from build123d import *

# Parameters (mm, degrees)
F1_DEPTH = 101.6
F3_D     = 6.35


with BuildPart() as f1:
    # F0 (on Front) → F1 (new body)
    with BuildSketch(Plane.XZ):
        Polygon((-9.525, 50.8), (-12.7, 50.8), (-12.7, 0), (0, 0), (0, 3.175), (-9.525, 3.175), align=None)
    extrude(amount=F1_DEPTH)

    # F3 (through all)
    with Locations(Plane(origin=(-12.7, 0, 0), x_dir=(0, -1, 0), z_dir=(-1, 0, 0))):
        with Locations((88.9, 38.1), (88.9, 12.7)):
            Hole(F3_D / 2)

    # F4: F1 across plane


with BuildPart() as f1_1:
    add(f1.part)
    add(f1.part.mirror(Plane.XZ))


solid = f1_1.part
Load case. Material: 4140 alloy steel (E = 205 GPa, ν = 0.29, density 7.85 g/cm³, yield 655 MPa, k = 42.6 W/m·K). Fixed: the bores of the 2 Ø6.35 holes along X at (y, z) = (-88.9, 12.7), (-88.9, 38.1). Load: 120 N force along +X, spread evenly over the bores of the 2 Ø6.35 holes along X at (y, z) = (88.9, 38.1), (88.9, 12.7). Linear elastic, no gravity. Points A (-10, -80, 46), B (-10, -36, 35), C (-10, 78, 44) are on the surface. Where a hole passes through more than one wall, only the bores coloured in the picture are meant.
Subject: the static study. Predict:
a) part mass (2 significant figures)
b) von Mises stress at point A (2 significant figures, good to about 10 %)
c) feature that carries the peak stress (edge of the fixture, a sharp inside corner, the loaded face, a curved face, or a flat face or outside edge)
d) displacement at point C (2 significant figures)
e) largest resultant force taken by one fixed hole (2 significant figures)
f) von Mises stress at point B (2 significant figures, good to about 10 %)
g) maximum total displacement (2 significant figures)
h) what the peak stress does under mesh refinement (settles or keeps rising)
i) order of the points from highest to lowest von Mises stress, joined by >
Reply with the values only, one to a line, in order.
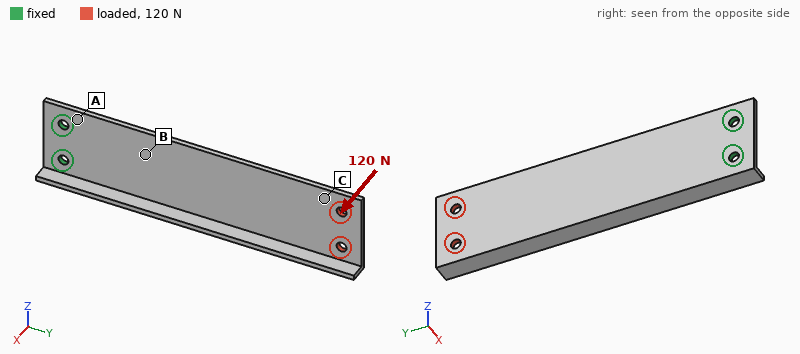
300 g
90 MPa
edge of the fixture
1.7 mm
160 N
31 MPa
2.1 mm
keeps rising
A > B > C
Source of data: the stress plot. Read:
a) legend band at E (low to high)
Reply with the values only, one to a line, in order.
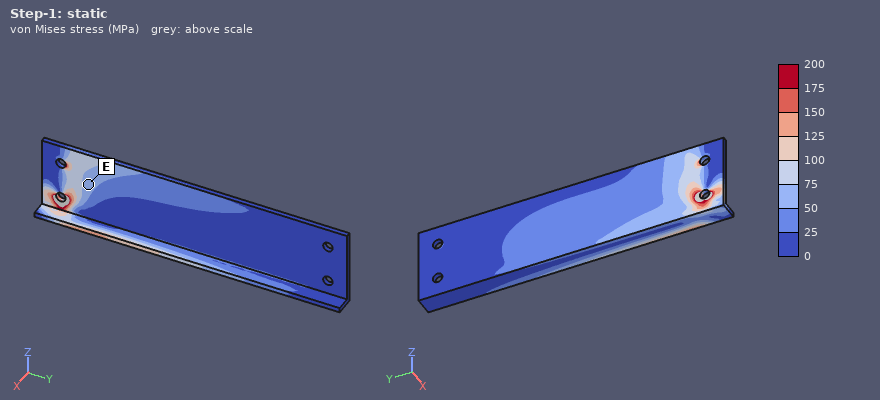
50 to 75 MPa
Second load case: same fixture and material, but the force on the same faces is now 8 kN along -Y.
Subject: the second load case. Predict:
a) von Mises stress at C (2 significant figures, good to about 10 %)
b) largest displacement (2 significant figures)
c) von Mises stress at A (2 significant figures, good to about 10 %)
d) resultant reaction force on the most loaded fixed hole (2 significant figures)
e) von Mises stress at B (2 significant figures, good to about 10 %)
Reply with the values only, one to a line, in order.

49 MPa
0.40 mm
41 MPa
4.0 kN
42 MPa
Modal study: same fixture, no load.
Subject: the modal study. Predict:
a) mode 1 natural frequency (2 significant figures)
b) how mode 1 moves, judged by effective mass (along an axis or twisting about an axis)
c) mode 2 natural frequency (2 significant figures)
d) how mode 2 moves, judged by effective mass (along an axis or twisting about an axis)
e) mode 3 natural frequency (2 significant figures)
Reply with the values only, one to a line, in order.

140 Hz
along X
510 Hz
twisting about Y
840 Hz
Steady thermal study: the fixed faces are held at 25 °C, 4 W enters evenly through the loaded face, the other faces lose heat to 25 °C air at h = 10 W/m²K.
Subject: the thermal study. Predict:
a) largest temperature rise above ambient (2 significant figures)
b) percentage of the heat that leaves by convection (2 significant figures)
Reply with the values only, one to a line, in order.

37 K
82 %
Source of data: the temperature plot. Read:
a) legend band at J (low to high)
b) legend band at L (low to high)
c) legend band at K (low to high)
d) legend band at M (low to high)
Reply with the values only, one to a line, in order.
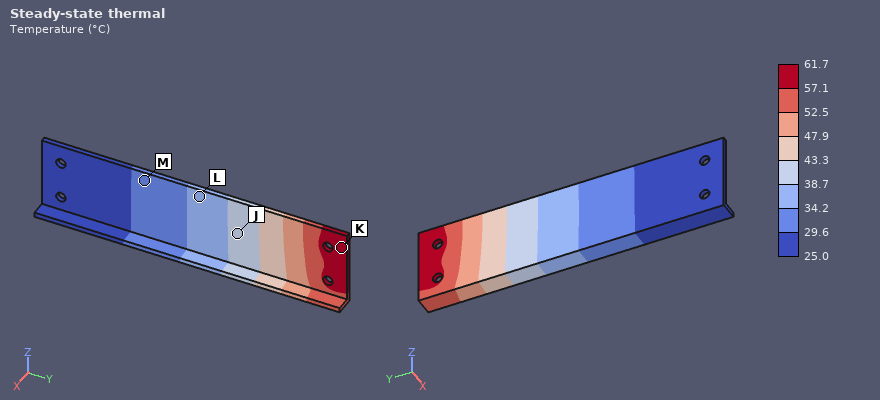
38.7 to 43.3 °C
34.2 to 38.7 °C
57.1 to 61.7 °C
29.6 to 34.2 °C
